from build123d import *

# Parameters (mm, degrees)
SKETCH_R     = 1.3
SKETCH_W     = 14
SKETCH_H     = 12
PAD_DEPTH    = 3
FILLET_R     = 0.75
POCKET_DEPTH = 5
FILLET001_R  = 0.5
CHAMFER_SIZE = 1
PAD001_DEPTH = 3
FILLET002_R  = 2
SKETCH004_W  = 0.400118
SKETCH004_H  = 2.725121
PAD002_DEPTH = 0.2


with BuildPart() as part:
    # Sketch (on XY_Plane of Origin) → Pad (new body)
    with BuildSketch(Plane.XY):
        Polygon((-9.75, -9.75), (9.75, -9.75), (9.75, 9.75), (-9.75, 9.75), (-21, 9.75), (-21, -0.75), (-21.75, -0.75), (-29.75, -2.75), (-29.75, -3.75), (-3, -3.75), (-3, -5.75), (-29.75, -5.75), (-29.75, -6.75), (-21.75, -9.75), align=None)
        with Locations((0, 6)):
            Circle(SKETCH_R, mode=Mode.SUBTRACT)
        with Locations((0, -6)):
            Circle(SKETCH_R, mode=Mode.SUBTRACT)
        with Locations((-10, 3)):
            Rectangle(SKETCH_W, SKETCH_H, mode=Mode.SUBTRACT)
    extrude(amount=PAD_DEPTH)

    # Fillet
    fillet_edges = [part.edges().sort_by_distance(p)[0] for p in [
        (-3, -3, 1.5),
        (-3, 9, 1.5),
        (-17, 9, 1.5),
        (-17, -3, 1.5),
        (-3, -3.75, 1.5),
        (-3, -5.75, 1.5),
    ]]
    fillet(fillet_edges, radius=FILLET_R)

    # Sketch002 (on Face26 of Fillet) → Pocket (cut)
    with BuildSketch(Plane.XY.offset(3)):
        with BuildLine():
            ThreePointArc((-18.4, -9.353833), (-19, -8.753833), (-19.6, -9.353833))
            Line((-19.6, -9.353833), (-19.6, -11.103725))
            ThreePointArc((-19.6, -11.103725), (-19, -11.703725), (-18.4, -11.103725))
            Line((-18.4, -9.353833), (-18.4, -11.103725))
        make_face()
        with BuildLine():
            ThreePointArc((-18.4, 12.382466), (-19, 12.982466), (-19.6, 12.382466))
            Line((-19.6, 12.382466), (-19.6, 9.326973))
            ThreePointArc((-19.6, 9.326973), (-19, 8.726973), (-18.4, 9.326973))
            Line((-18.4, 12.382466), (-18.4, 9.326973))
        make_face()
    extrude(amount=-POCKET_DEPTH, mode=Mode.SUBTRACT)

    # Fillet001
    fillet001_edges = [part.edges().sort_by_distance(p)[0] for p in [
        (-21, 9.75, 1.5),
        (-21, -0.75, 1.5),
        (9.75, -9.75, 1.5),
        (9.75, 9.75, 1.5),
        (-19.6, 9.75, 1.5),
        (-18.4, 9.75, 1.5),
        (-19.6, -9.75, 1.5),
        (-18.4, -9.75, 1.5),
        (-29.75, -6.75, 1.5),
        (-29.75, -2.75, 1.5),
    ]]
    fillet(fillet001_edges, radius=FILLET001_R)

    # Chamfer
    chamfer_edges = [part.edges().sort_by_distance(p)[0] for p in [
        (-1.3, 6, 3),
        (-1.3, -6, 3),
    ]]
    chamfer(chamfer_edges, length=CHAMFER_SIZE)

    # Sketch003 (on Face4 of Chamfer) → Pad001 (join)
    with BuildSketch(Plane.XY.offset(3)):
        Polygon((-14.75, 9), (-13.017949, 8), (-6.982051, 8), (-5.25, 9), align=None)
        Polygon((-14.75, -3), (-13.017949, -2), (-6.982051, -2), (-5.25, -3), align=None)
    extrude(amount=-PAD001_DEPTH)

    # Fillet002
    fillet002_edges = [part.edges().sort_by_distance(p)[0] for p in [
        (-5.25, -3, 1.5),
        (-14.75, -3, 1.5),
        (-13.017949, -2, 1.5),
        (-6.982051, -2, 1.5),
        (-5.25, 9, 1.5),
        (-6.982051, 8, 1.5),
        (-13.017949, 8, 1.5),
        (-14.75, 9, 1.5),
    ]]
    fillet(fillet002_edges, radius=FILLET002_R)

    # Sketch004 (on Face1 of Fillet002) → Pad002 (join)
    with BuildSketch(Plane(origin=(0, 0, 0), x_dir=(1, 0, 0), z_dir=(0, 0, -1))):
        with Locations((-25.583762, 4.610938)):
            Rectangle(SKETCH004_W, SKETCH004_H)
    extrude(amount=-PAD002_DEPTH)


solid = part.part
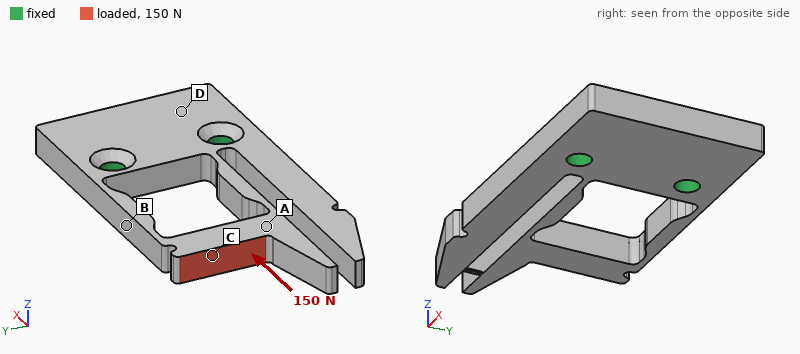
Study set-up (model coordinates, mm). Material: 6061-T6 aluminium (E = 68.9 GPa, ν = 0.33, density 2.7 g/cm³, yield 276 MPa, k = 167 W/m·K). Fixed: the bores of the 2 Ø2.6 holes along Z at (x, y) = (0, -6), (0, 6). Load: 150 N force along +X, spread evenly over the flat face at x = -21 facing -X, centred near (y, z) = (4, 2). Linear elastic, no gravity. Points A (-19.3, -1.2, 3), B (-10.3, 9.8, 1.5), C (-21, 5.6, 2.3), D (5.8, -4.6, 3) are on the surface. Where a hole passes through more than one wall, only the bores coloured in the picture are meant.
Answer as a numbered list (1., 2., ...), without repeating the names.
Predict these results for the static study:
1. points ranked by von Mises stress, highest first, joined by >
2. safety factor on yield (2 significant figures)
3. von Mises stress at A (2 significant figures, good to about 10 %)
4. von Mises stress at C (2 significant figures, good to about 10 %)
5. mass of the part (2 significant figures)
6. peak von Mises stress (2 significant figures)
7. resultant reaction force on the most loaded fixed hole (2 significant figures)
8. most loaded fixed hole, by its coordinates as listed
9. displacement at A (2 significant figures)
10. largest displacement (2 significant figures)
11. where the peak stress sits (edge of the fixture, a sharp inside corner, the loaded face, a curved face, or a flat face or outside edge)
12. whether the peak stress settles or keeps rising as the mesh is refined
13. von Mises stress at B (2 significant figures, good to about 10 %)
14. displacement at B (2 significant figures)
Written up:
1. B > C > A > D
2. 2.9
3. 14 MPa
4. 25 MPa
5. 3.5 g
6. 94 MPa
7. 120 N
8. (0, 6)
9. 9.1 µm
10. 14 µm
11. a curved face
12. settles
13. 40 MPa
14. 6.7 µm
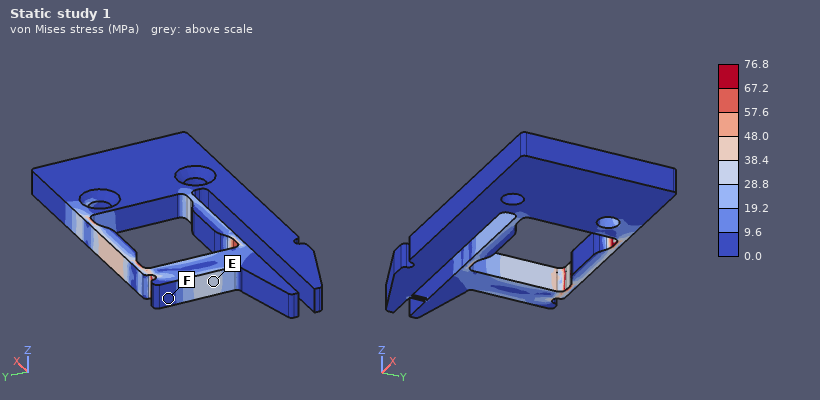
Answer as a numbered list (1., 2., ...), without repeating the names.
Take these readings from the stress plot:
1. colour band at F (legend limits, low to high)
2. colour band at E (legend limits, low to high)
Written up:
1. 0.0 to 9.6 MPa
2. 28.8 to 38.4 MPa
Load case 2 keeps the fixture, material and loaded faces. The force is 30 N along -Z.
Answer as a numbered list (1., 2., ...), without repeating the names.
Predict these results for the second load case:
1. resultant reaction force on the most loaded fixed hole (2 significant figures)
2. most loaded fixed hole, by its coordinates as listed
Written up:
1. 17 N
2. (0, 6)
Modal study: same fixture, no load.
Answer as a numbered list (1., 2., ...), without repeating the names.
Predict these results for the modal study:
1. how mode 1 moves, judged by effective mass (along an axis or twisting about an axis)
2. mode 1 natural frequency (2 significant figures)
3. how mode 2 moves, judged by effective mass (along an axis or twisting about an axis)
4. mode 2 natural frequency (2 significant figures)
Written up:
1. along Z
2. 2500 Hz
3. along Y
4. 2800 Hz
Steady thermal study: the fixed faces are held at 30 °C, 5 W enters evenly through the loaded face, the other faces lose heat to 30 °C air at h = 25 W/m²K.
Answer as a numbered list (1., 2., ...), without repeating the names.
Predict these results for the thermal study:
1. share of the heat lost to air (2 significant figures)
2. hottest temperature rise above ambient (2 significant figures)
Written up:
1. 12 %
2. 66 K
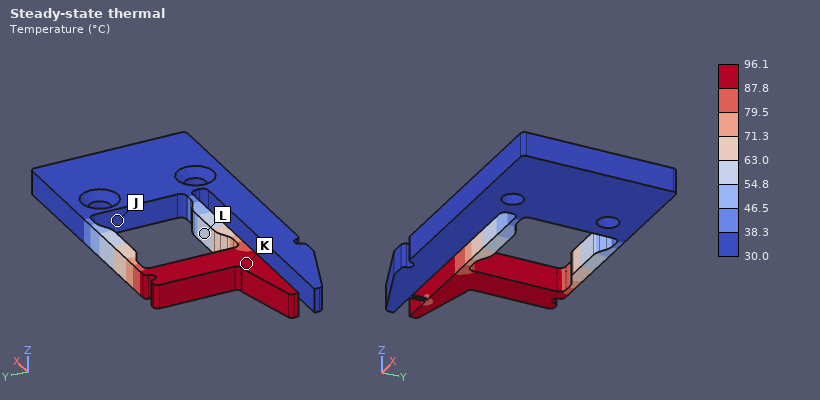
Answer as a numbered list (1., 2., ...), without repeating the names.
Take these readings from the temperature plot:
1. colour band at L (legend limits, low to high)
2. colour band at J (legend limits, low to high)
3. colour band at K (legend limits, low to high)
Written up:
1. 54.8 to 63.0 °C
2. 30.0 to 38.3 °C
3. 87.8 to 96.1 °C
